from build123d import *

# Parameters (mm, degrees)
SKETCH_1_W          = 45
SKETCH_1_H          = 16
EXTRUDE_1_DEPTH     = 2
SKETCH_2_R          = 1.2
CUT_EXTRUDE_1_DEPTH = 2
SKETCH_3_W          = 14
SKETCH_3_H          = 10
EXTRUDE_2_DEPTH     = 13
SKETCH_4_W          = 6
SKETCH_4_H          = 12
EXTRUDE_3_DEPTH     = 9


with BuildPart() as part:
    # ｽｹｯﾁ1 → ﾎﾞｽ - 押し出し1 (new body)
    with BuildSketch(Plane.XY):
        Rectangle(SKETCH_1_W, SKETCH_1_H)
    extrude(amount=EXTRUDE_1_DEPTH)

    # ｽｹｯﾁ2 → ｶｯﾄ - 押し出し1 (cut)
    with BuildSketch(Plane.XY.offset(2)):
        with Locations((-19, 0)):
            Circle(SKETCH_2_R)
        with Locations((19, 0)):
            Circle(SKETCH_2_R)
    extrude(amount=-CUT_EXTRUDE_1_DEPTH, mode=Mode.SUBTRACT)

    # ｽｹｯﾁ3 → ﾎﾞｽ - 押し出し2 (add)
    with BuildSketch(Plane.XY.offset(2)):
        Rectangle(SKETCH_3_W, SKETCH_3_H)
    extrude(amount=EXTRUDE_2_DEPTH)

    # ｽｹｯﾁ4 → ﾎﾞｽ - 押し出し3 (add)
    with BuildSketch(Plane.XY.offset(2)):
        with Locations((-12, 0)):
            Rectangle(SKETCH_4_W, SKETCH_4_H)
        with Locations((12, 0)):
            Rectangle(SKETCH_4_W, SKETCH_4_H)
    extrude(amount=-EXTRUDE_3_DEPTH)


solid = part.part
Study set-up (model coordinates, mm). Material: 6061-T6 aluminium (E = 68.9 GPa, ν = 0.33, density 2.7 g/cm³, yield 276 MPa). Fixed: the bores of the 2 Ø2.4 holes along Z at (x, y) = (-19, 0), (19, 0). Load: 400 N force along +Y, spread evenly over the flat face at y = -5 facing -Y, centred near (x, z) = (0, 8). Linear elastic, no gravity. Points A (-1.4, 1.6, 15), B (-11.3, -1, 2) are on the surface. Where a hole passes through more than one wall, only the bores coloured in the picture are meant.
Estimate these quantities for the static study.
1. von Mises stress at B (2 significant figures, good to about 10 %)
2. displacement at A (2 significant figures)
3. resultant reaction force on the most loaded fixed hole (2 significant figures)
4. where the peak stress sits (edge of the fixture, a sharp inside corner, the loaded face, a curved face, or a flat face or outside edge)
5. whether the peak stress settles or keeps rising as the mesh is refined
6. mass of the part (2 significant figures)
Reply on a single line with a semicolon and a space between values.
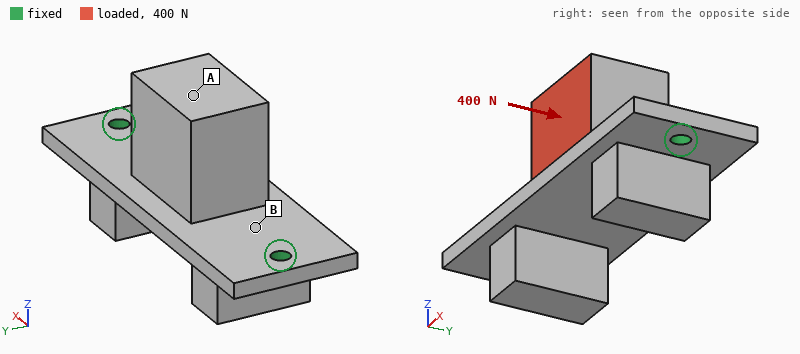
48 MPa; 0.13 mm; 200 N; edge of the fixture; keeps rising; 11 g
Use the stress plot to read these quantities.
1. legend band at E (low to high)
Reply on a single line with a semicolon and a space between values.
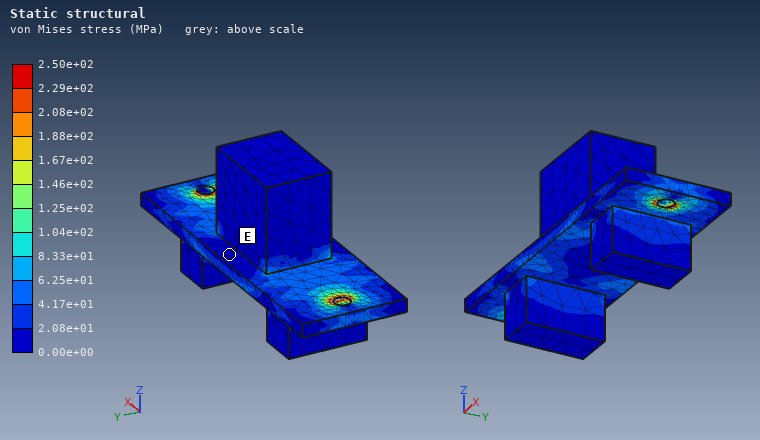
0.00e+00 to 2.08e+01 MPa
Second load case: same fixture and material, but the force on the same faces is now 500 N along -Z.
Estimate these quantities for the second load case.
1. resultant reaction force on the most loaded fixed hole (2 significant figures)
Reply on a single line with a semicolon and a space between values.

270 N
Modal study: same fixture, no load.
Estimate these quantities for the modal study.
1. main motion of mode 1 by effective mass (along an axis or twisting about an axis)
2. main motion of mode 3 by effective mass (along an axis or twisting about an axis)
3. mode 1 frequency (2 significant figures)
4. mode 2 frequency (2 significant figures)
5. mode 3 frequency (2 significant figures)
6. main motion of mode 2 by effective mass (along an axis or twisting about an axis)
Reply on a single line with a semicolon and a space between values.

along Y; along X; 4200 Hz; 4500 Hz; 7300 Hz; along Z
